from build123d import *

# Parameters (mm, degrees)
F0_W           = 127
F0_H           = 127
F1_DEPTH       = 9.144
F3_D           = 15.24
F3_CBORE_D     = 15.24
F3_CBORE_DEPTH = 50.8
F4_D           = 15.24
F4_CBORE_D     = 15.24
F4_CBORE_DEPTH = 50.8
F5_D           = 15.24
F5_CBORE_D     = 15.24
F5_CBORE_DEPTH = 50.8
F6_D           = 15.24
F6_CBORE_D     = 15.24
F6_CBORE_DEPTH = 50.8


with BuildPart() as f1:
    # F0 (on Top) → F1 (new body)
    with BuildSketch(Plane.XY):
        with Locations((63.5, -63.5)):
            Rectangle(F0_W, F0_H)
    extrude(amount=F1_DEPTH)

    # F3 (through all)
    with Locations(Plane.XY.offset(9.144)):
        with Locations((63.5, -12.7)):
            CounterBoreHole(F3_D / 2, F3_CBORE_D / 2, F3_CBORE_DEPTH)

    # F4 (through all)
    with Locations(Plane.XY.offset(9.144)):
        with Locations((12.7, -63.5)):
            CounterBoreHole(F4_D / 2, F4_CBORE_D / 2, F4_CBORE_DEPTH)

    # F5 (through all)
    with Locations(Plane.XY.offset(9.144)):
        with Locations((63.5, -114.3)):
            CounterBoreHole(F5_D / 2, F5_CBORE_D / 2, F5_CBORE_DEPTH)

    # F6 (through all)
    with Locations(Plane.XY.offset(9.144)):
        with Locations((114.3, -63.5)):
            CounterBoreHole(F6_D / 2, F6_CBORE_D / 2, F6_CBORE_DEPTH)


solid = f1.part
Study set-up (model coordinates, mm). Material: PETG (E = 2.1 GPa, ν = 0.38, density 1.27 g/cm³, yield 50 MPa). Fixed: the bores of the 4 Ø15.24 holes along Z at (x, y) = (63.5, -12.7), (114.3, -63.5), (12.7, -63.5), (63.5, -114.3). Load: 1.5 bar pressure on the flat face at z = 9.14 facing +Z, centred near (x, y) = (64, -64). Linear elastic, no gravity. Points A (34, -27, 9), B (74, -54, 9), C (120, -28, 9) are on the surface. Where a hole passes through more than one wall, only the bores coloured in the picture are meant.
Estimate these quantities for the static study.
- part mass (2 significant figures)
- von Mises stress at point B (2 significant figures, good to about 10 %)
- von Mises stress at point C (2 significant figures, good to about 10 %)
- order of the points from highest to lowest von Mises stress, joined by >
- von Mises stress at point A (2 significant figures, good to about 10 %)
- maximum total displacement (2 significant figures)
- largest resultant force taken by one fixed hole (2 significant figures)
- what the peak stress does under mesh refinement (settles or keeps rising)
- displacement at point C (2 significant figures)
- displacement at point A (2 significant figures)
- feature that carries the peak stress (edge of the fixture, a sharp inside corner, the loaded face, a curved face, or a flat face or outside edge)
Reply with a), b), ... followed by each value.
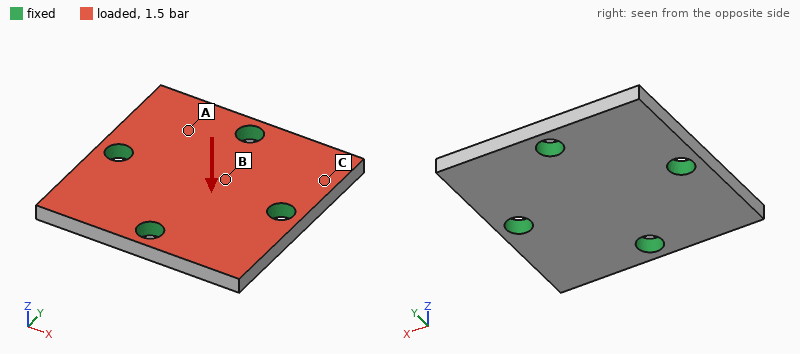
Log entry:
a) 180 g
b) 0.97 MPa
c) 2.6 MPa
d) A > C > B
e) 3.3 MPa
f) 0.55 mm
g) 580 N
h) keeps rising
i) 0.24 mm
j) 0.12 mm
k) edge of the fixture
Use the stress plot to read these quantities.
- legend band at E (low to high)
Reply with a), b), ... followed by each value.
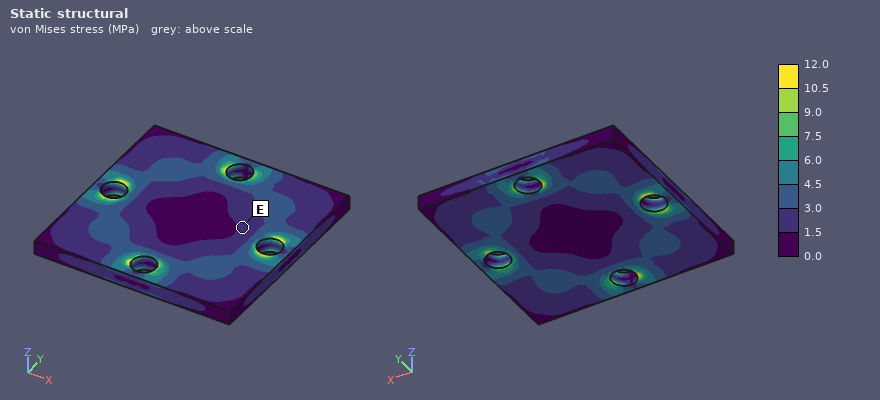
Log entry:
a) 1.5 to 3.0 MPa
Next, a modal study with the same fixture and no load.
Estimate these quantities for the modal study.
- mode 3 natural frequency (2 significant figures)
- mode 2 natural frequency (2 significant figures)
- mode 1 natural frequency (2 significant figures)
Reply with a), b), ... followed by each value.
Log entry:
a) 1100 Hz
b) 1100 Hz
c) 1100 Hz
